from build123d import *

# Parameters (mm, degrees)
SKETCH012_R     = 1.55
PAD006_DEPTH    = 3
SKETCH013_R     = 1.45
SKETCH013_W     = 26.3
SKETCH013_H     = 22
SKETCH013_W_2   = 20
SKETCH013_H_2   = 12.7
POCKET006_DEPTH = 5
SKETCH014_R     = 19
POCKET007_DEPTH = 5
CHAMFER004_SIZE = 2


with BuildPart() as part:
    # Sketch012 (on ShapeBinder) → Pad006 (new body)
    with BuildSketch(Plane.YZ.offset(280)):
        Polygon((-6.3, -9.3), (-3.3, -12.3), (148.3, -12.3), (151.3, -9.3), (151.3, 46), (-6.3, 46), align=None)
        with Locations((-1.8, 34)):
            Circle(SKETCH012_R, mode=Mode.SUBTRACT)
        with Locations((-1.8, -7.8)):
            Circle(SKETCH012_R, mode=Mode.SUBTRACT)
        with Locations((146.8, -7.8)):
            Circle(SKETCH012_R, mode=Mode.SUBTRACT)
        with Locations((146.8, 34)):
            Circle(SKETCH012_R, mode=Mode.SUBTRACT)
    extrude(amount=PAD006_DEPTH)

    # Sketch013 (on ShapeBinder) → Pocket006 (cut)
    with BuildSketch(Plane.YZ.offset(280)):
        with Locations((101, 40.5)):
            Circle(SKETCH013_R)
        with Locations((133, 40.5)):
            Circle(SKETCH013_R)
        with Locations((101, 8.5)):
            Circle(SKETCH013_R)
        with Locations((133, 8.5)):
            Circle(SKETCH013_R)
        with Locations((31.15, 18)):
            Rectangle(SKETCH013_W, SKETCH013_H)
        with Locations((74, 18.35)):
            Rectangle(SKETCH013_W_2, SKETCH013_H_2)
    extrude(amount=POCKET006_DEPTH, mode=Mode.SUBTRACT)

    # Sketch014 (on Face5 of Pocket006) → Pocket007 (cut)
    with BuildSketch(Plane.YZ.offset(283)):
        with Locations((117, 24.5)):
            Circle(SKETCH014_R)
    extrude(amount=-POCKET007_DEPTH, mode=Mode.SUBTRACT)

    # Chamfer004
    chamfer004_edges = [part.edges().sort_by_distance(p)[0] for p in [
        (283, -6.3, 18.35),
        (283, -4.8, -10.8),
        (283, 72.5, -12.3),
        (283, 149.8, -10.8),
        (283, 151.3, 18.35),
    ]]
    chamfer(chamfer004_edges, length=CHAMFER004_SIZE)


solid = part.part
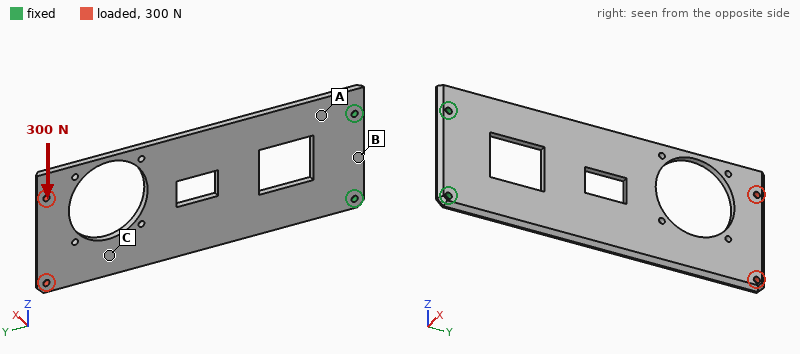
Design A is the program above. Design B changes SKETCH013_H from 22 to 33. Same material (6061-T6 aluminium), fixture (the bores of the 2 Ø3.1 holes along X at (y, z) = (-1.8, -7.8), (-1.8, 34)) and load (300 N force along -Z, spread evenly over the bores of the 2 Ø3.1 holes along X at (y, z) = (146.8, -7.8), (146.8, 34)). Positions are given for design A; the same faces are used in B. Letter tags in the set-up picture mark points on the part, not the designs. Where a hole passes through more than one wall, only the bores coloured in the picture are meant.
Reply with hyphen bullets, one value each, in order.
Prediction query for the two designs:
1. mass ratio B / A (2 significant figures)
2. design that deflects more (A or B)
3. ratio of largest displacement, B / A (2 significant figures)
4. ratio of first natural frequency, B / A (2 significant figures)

- 0.96
- B
- 1.2
- 0.89
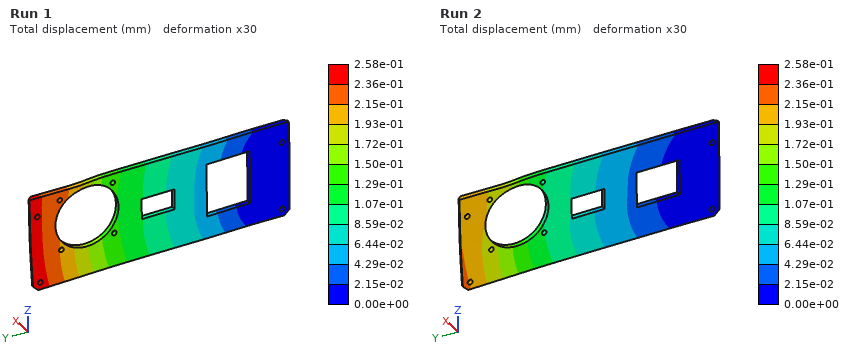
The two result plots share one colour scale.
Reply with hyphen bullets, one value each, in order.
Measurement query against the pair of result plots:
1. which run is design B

- Run 1
